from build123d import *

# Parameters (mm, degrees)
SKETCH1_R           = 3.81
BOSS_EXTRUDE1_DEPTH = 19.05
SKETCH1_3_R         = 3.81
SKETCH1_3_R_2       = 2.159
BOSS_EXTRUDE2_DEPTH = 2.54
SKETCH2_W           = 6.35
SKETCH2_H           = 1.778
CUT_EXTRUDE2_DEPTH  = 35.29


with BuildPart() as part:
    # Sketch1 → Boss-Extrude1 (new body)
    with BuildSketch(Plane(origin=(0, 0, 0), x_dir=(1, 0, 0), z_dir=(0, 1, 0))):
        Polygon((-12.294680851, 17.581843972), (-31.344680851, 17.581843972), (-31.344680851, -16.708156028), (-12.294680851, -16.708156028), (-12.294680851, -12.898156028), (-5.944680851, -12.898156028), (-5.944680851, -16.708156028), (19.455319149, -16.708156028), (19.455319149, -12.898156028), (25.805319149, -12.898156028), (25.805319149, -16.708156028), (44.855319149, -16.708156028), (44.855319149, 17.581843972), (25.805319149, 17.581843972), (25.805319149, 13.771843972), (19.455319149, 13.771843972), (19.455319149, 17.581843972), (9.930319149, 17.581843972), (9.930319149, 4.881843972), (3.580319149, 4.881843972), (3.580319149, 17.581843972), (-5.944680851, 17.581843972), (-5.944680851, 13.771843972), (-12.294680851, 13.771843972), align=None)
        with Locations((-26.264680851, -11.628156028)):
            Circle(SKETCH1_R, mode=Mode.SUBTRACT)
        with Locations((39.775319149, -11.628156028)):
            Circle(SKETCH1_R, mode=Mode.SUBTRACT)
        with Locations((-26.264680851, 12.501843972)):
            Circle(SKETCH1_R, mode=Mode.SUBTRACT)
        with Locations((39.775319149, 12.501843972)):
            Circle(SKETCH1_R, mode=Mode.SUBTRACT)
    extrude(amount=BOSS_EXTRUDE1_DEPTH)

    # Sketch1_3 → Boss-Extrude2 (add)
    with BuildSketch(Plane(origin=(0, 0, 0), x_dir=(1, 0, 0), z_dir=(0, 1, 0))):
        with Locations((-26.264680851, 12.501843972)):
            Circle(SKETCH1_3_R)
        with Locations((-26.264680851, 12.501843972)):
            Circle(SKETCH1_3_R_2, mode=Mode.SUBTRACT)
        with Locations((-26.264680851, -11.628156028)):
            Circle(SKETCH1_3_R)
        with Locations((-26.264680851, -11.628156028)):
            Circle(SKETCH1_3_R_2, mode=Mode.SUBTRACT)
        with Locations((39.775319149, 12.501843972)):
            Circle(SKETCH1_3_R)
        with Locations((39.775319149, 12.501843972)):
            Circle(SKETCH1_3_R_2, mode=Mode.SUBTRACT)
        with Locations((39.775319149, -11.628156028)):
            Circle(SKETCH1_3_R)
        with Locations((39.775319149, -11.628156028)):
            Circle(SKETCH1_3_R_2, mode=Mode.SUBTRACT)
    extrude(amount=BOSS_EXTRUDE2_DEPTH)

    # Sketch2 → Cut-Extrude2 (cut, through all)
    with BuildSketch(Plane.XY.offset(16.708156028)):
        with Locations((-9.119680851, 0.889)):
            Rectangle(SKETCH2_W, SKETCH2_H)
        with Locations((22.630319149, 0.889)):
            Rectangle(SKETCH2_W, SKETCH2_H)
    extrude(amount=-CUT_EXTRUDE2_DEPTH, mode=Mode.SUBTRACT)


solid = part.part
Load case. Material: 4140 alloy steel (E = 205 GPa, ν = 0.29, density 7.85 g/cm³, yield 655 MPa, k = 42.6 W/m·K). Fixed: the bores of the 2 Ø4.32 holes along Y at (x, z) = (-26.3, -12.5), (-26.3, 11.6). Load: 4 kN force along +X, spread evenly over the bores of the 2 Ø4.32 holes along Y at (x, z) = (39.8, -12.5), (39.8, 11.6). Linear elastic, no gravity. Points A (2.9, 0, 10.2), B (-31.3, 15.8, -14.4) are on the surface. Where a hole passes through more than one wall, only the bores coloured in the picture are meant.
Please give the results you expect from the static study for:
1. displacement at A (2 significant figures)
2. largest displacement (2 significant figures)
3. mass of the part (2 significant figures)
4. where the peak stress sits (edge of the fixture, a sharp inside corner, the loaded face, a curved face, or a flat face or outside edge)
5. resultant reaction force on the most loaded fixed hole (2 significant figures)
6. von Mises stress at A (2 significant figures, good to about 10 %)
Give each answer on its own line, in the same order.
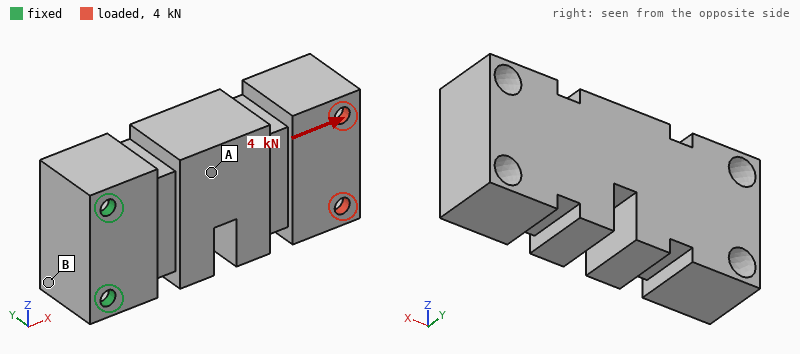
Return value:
6.8 µm
35 µm
330 g
the loaded face
2.0 kN
23 MPa
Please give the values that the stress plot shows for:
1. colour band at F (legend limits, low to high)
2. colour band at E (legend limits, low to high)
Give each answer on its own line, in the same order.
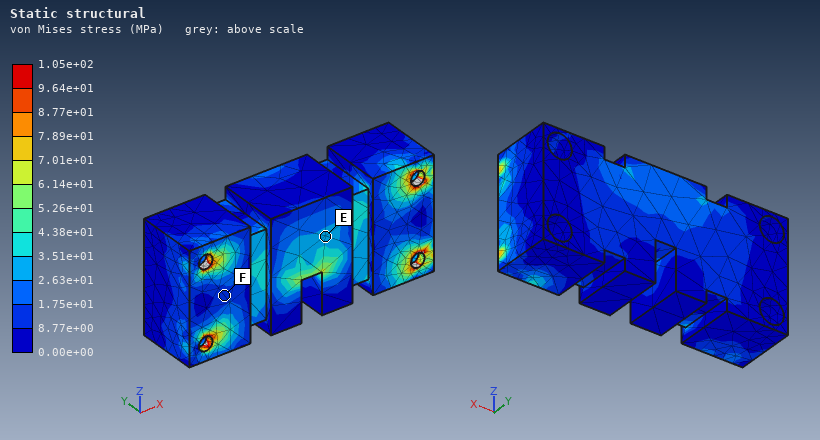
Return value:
8.77e+00 to 1.75e+01 MPa
2.63e+01 to 3.51e+01 MPa
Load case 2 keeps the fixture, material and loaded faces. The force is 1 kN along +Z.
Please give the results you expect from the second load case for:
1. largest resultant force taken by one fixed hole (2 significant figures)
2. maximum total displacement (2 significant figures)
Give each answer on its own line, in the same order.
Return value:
2.6 kN
44 µm
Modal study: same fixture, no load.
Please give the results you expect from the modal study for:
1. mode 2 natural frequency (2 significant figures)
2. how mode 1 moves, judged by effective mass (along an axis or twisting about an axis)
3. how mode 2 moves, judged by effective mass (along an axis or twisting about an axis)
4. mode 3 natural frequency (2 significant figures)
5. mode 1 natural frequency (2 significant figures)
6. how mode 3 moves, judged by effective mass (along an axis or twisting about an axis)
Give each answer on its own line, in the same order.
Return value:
2700 Hz
along Y
along Z
6700 Hz
720 Hz
twisting about X
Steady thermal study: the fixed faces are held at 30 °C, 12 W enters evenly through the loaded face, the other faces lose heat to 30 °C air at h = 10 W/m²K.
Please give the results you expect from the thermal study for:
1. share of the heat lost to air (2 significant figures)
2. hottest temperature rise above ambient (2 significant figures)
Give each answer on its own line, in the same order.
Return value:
24 %
57 K
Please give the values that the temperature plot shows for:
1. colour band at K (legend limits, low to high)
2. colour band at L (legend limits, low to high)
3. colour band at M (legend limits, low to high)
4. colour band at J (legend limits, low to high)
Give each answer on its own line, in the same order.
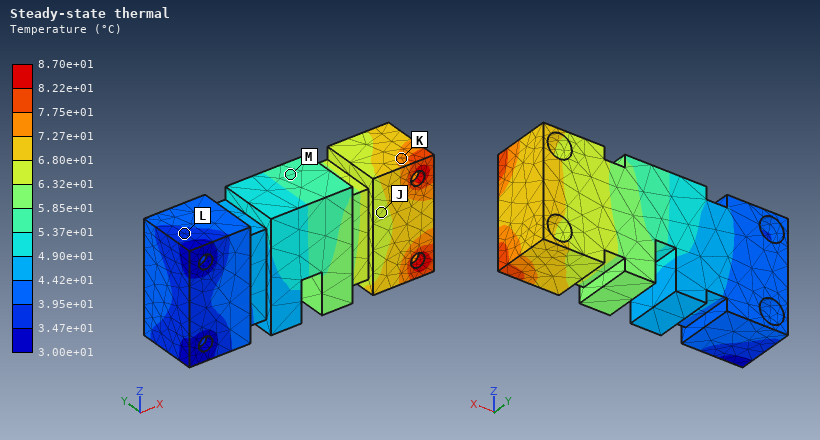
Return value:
7.27e+01 to 7.75e+01 °C
3.47e+01 to 3.95e+01 °C
5.37e+01 to 5.85e+01 °C
6.32e+01 to 6.80e+01 °C
